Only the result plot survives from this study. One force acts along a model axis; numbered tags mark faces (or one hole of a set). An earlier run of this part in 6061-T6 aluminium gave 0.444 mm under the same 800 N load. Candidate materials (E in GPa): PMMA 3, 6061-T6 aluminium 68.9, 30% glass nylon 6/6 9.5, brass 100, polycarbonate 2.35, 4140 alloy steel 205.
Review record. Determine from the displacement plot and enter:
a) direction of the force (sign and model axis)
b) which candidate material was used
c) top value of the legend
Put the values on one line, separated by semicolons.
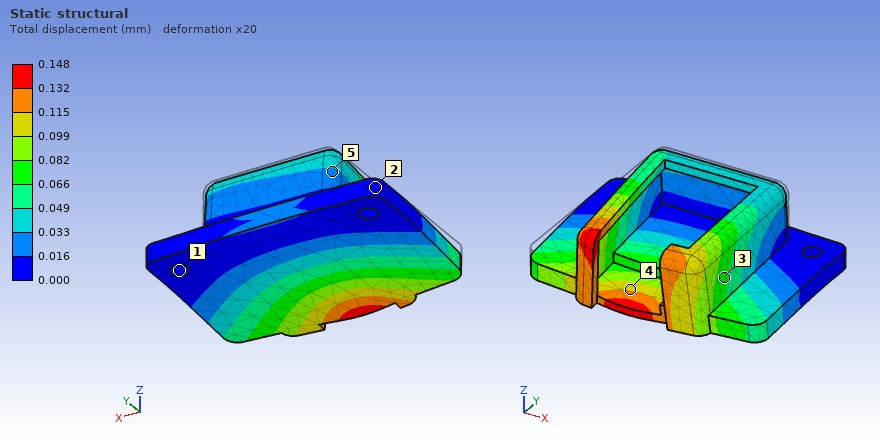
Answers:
-Z; 4140 alloy steel; 0.148 mm
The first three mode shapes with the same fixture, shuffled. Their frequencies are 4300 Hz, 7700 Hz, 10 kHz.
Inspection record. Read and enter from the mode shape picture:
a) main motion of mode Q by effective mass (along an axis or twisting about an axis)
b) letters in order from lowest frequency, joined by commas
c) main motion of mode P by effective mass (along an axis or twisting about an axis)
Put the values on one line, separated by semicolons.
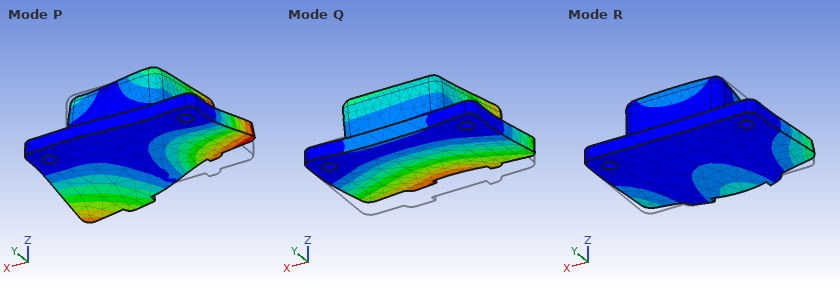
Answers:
along Z; Q, P, R; twisting about Y
